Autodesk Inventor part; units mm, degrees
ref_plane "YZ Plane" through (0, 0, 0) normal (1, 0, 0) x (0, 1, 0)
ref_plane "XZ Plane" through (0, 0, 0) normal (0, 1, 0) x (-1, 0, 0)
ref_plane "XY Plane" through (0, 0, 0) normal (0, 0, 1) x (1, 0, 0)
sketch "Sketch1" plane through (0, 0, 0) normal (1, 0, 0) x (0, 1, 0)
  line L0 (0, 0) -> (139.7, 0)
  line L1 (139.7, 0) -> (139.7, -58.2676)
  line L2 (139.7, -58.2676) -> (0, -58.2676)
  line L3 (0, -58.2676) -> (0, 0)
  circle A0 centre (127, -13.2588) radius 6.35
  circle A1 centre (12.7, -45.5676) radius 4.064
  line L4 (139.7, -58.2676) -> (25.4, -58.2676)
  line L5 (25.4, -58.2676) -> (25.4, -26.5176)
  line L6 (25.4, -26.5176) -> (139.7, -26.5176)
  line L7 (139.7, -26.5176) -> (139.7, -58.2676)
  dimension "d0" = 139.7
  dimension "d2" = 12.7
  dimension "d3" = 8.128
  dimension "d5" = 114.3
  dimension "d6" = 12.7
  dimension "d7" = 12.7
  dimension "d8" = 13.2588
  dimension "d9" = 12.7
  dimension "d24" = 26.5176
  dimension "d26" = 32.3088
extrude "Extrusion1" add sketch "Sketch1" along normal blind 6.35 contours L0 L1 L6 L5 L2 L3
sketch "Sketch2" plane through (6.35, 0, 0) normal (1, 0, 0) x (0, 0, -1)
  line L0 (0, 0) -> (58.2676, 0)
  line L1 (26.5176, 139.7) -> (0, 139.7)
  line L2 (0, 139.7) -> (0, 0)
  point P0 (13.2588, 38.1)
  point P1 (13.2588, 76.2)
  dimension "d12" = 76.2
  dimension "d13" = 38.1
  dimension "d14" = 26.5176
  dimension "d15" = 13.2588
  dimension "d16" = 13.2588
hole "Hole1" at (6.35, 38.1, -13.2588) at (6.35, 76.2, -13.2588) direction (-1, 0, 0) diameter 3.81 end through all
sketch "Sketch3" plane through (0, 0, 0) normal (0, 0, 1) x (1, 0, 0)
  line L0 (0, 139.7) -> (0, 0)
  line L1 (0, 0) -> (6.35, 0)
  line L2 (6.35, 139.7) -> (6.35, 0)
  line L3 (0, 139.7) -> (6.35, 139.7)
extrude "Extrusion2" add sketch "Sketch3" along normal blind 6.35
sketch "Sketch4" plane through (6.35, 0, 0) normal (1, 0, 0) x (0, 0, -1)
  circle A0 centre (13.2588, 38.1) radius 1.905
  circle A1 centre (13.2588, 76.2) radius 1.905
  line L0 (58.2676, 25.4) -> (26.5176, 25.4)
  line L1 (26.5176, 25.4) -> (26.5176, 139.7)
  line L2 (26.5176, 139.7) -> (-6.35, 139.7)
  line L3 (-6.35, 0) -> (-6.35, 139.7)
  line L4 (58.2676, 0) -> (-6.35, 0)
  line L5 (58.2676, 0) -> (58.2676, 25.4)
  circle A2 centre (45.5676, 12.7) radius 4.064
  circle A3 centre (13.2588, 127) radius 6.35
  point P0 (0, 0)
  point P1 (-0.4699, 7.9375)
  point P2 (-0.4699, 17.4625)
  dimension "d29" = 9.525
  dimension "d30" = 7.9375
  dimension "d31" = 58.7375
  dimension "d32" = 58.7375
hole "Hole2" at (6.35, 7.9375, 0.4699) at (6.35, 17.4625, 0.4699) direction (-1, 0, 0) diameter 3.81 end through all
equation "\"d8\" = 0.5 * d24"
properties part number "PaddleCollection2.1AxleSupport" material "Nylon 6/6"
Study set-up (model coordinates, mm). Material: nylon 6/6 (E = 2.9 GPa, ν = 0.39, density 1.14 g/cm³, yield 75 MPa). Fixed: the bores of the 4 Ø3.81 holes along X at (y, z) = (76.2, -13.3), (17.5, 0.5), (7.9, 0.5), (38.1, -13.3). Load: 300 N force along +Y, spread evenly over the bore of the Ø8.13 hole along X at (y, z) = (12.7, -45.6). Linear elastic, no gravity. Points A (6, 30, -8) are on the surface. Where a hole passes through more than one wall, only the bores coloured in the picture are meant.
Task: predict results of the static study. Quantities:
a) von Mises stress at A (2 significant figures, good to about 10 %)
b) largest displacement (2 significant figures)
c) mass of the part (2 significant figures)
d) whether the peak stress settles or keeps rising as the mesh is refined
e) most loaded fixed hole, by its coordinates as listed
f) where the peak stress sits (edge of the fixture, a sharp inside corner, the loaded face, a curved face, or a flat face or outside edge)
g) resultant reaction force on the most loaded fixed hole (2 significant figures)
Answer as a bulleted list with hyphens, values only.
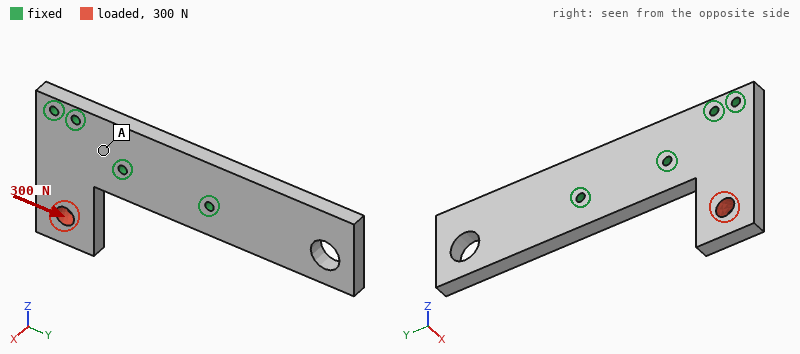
- 1.4 MPa
- 0.29 mm
- 37 g
- keeps rising
- (38.1, -13.3)
- a sharp inside corner
- 370 N
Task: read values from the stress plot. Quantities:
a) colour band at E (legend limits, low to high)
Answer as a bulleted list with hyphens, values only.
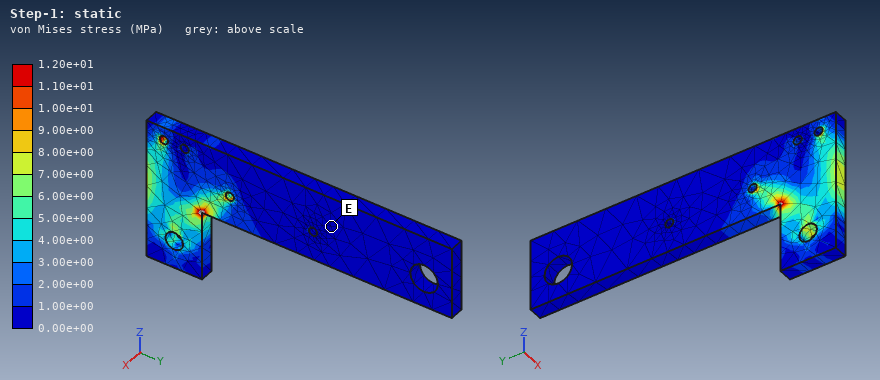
- 0.00e+00 to 1.00e+00 MPa
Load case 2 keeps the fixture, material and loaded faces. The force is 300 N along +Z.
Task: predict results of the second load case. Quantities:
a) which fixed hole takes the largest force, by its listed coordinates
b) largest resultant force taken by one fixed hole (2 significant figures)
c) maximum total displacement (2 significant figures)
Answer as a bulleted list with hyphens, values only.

- (7.9, 0.5)
- 170 N
- 44 µm
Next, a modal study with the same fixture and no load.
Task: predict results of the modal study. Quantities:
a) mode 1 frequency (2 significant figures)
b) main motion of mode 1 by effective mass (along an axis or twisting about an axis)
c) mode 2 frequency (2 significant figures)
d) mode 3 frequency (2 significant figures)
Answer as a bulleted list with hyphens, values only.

- 410 Hz
- along X
- 660 Hz
- 1300 Hz
